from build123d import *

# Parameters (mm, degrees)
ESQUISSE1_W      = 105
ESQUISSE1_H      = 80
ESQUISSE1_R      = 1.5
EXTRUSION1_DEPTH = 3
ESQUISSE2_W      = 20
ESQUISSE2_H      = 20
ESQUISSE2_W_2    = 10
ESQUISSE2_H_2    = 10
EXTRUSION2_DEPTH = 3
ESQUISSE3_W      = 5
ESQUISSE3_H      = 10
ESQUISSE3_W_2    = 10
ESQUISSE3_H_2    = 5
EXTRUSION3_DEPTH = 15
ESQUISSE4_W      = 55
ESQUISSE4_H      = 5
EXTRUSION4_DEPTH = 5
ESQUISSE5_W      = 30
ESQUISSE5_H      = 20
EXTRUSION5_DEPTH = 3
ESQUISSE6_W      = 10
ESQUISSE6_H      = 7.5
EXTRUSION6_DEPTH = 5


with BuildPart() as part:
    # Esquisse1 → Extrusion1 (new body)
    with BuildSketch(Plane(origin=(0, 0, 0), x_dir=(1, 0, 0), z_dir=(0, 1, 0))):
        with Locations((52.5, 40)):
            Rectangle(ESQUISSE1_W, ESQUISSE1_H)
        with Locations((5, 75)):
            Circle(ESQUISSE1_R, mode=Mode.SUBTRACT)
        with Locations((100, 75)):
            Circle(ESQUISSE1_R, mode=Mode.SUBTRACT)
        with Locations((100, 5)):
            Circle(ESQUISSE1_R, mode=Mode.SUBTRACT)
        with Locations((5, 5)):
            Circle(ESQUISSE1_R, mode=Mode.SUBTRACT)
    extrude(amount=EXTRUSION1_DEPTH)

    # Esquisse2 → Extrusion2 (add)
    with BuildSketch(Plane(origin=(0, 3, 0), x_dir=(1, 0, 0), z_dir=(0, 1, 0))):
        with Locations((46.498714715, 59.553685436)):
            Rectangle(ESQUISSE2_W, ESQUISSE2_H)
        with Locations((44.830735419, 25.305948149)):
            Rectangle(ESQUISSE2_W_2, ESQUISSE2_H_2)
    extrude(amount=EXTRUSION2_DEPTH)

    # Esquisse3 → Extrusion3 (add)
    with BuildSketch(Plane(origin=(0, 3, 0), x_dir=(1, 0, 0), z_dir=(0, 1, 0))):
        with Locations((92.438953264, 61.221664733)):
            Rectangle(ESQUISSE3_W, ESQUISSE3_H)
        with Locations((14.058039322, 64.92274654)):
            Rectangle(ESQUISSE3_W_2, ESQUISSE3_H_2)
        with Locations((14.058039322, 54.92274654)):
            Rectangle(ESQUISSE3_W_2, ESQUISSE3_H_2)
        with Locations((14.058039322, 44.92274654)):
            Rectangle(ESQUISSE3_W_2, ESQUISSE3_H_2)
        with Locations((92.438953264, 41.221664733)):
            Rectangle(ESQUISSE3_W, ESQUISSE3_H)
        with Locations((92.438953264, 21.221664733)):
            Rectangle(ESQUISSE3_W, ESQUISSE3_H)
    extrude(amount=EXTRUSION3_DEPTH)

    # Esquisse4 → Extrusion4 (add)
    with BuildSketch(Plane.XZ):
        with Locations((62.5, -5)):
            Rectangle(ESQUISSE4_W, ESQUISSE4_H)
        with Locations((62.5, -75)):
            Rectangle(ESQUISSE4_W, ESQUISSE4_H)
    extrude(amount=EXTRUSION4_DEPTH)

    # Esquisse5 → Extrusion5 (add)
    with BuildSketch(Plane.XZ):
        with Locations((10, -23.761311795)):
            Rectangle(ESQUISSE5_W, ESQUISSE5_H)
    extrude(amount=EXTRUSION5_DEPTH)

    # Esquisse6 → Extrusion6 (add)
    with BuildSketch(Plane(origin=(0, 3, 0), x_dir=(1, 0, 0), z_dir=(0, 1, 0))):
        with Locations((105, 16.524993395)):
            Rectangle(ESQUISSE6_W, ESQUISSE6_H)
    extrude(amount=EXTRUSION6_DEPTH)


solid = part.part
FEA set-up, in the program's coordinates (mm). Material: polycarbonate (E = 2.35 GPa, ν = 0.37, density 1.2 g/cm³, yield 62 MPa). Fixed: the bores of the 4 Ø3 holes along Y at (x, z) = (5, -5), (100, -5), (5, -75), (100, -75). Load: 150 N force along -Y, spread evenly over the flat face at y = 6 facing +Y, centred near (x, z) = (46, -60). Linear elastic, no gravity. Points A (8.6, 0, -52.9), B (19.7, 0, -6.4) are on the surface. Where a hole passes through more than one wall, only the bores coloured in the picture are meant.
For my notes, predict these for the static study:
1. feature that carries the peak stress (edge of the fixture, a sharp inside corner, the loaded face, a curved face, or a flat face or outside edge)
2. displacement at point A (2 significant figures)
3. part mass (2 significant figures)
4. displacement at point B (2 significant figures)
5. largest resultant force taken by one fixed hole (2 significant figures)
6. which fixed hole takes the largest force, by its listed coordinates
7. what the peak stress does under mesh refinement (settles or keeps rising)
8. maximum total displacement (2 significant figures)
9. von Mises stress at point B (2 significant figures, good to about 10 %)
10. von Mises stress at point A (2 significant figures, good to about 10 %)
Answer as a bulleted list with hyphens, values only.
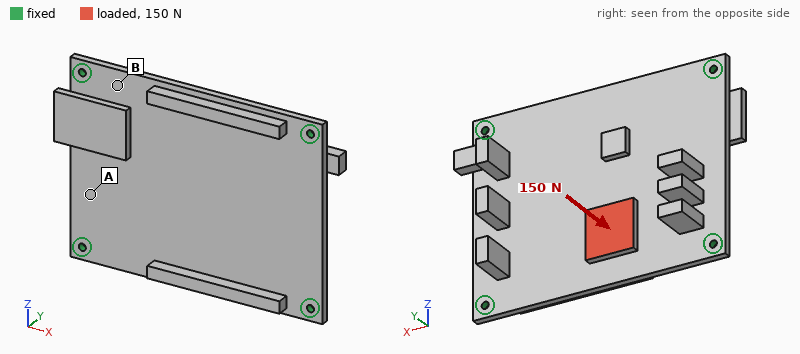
- edge of the fixture
- 0.44 mm
- 43 g
- 0.25 mm
- 80 N
- (5, -75)
- keeps rising
- 1.5 mm
- 2.0 MPa
- 4.0 MPa
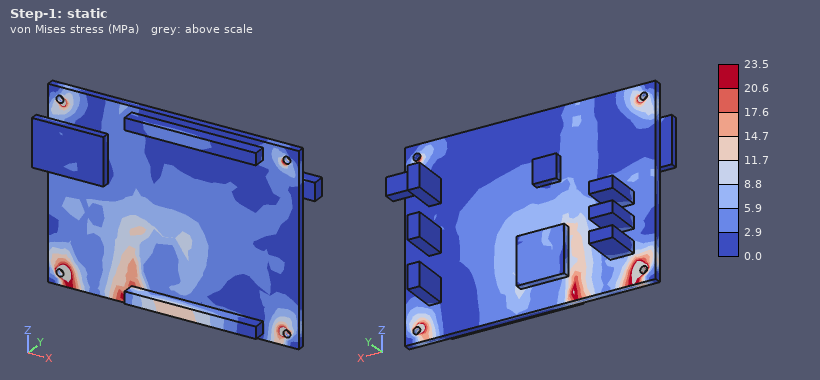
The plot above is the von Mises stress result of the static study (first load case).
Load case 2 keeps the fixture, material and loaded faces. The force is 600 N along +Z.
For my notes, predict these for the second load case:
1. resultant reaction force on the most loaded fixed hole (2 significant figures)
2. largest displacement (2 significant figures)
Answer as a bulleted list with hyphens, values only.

- 200 N
- 0.90 mm
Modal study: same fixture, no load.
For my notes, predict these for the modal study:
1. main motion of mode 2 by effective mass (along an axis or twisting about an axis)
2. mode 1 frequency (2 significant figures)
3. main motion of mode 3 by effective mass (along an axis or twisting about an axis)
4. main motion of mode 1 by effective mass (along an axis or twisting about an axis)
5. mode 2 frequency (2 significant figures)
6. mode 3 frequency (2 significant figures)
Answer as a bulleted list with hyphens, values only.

- twisting about X
- 400 Hz
- twisting about Z
- along Y
- 680 Hz
- 740 Hz
